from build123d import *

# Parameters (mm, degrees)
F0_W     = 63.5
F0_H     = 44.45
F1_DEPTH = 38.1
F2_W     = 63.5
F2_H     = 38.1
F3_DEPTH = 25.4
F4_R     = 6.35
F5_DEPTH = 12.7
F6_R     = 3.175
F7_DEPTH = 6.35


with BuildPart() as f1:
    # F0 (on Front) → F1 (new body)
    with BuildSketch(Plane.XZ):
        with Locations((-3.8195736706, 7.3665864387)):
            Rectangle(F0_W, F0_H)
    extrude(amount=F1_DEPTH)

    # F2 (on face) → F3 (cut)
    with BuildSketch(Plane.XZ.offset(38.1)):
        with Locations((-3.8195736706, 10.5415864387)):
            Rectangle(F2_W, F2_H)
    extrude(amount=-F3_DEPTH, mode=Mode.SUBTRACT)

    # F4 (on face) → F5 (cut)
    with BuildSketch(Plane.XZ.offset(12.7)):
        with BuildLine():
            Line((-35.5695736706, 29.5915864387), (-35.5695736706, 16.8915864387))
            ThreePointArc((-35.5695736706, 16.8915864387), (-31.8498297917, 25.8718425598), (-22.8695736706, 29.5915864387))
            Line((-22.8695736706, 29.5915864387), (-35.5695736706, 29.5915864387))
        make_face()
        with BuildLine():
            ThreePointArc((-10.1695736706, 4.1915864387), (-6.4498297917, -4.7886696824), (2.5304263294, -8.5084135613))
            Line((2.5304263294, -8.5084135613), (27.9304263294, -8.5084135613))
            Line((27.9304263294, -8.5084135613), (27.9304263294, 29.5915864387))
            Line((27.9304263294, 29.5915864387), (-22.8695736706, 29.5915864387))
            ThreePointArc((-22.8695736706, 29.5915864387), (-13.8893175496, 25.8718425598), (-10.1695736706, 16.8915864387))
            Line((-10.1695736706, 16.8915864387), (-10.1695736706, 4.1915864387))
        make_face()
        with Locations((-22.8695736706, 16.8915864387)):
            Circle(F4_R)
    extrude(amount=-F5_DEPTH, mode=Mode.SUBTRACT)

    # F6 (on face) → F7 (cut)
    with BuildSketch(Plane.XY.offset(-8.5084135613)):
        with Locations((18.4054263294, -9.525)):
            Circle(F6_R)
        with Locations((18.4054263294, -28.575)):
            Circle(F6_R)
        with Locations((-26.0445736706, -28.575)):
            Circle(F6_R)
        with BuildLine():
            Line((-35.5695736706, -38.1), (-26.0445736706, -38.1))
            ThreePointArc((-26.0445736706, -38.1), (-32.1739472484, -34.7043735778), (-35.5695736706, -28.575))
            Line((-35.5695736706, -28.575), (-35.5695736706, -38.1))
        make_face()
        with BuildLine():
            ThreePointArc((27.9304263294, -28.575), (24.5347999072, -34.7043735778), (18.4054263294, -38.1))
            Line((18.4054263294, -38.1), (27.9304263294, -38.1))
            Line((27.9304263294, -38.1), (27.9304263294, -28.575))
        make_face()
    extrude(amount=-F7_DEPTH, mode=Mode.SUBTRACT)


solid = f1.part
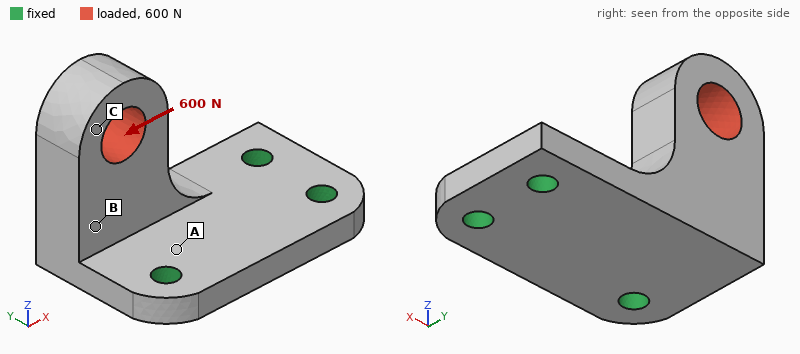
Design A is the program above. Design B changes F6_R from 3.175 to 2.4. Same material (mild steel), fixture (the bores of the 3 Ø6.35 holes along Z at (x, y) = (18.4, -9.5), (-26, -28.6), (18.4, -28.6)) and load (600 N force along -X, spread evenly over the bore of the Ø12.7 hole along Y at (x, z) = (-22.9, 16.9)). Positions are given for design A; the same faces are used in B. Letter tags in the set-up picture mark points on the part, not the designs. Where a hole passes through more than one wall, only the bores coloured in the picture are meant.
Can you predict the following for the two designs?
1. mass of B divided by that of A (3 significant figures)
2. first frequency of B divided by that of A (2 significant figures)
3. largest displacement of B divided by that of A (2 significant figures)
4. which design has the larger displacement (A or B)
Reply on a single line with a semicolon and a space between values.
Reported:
1.01; 0.96; 1.1; B
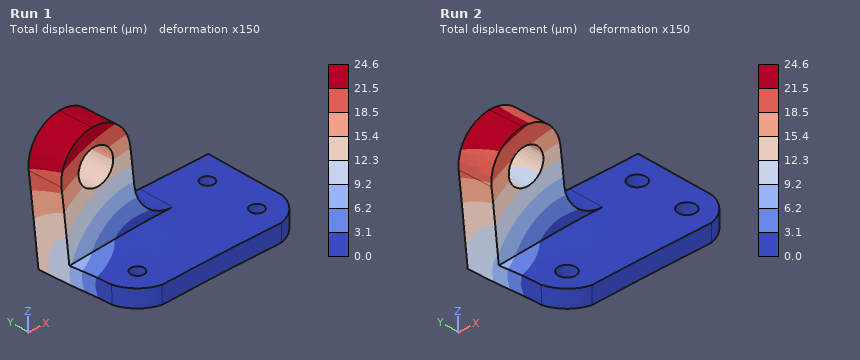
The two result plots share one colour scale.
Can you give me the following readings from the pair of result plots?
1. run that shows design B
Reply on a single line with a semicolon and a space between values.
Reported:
Run 1
